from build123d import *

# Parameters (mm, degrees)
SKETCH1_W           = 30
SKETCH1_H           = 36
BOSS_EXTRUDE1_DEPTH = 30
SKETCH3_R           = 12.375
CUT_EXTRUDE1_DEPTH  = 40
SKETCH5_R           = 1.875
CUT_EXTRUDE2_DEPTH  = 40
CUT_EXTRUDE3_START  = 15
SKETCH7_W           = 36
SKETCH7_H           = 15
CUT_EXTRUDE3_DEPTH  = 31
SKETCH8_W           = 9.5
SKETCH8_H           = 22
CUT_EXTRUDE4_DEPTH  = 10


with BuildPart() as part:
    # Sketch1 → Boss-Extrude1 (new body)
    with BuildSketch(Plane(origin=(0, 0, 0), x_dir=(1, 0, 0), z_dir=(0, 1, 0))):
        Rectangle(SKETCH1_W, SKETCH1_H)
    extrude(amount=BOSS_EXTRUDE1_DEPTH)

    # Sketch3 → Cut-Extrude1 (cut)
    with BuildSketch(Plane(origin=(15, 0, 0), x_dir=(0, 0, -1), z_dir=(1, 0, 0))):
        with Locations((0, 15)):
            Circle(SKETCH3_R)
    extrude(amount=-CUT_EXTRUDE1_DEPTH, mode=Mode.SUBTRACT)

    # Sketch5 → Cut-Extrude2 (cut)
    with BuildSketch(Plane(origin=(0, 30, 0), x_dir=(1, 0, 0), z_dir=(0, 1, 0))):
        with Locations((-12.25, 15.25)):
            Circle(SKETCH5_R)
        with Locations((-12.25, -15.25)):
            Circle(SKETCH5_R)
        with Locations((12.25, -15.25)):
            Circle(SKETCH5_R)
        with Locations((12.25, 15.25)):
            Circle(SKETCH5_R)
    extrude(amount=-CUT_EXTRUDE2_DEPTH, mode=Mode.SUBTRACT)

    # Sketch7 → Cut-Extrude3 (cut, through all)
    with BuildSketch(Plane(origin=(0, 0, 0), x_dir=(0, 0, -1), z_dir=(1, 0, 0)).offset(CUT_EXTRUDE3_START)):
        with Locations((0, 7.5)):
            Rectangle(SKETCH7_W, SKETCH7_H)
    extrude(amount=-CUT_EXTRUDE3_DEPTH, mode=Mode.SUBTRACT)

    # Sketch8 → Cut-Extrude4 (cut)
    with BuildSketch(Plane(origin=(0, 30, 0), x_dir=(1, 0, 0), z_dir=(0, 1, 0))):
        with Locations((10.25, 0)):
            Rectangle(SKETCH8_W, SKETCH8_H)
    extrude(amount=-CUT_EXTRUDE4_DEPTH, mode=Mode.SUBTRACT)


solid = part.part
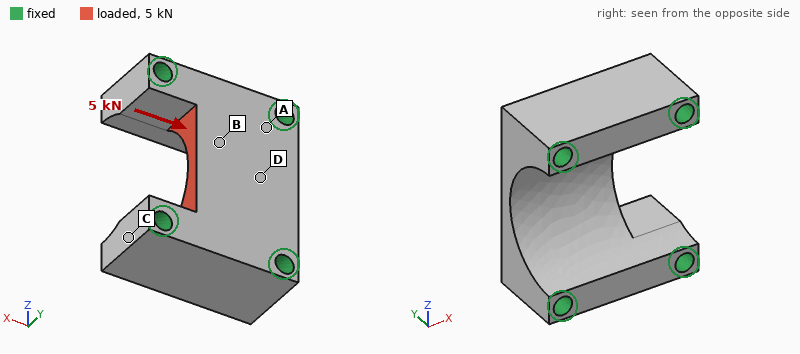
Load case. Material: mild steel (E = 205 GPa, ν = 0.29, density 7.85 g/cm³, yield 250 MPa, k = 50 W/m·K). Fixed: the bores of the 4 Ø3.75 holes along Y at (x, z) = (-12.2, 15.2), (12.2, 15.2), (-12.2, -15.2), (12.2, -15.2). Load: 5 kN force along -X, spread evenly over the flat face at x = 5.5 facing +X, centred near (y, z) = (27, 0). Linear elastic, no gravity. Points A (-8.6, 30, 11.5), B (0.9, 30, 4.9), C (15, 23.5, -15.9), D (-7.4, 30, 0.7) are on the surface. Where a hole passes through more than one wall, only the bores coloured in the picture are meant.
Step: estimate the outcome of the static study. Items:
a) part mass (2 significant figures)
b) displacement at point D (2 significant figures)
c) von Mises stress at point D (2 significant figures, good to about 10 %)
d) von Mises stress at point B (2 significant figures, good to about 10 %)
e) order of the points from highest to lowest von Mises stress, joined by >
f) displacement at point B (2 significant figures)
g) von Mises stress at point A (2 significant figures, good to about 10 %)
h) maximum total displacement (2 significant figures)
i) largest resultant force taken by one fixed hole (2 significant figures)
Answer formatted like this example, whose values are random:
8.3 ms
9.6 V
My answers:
58 g
2.5 µm
17 MPa
47 MPa
B > A > D > C
3.3 µm
34 MPa
5.2 µm
1.7 kN
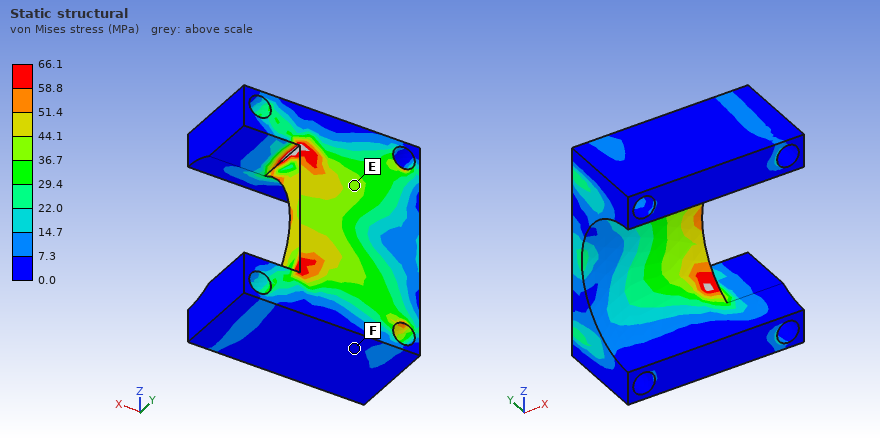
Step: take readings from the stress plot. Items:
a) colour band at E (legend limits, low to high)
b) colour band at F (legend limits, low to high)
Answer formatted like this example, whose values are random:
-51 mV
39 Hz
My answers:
36.7 to 44.1 MPa
0.0 to 7.3 MPa
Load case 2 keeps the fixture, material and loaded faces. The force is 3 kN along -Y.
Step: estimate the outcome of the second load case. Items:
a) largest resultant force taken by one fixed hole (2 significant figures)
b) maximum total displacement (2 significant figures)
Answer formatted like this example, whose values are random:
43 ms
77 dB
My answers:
1.2 kN
18 µm
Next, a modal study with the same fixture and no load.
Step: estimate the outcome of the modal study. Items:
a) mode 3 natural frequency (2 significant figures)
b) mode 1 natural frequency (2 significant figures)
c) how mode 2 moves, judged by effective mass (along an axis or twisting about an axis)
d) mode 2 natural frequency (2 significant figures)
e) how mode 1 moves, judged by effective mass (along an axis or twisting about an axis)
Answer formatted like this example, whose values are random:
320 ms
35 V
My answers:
50 kHz
37 kHz
along Z
45 kHz
along Y
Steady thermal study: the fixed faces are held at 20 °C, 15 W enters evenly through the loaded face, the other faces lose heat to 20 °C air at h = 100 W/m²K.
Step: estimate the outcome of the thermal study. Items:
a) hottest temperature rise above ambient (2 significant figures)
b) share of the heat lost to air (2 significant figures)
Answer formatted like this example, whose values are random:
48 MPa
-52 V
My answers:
27 K
8.5 %
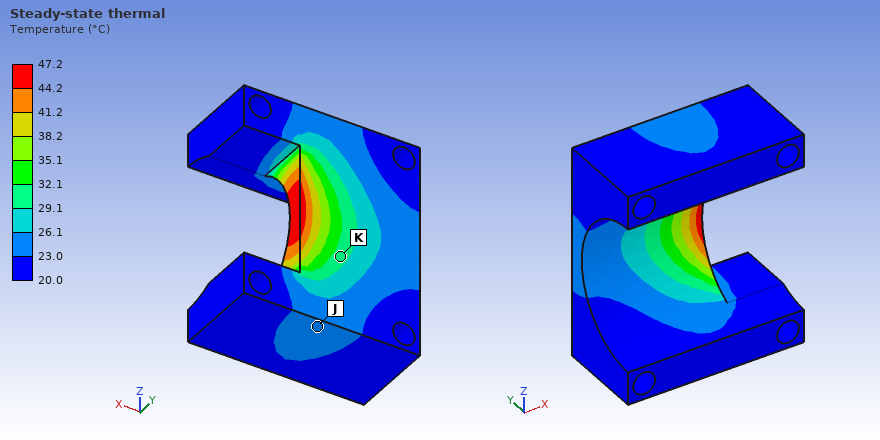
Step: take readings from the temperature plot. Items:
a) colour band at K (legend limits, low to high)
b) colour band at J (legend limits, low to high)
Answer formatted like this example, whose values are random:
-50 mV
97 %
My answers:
29.1 to 32.1 °C
23.0 to 26.1 °C
